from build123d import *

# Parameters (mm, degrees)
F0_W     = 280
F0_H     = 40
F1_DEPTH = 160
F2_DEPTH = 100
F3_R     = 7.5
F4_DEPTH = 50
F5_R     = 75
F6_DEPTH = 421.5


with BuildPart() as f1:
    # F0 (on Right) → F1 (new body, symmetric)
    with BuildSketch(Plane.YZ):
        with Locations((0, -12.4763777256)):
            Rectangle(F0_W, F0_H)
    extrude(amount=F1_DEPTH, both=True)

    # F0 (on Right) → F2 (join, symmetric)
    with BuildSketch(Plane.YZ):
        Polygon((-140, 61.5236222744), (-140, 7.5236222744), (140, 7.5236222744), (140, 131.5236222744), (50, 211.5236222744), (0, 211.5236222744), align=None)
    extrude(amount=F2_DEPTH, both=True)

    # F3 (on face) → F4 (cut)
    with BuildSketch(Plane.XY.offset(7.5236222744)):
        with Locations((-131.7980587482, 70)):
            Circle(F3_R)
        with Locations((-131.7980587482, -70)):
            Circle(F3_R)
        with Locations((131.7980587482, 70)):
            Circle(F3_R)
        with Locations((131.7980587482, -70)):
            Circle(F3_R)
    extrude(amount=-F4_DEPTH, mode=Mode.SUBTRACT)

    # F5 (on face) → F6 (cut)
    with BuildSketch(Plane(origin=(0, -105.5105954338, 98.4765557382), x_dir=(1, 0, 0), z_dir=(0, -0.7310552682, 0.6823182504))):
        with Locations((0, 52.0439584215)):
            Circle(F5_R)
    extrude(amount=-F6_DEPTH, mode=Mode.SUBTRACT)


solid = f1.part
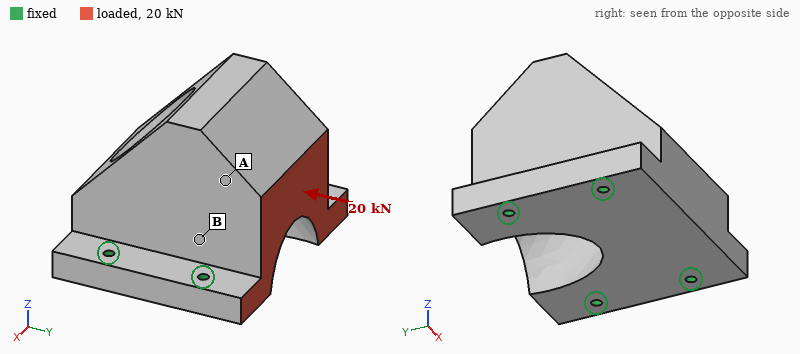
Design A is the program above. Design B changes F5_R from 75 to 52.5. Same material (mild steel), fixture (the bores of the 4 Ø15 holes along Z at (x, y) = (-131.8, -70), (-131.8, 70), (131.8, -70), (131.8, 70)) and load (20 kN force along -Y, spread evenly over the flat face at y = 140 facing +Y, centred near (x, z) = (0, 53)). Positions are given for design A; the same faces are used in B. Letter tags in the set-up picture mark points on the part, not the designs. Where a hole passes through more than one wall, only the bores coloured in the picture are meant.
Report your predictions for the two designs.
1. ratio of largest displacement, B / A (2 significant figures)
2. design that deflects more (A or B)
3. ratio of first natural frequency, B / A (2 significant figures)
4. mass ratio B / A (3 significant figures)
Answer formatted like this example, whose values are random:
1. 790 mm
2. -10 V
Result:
1. 0.78
2. A
3. 0.96
4. 1.25
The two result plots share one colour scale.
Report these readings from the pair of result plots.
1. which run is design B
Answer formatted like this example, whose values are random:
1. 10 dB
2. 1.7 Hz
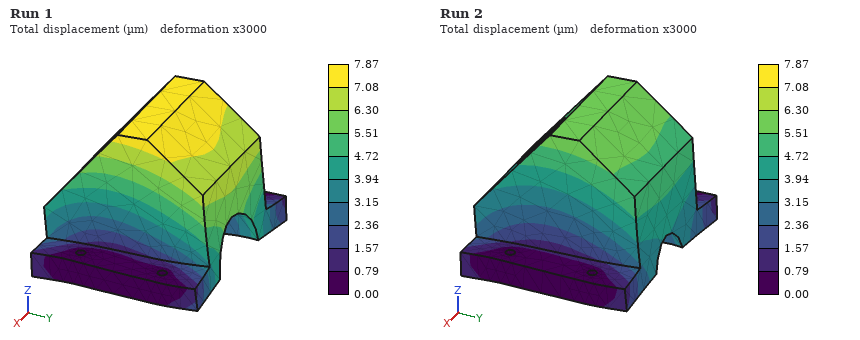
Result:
1. Run 2
